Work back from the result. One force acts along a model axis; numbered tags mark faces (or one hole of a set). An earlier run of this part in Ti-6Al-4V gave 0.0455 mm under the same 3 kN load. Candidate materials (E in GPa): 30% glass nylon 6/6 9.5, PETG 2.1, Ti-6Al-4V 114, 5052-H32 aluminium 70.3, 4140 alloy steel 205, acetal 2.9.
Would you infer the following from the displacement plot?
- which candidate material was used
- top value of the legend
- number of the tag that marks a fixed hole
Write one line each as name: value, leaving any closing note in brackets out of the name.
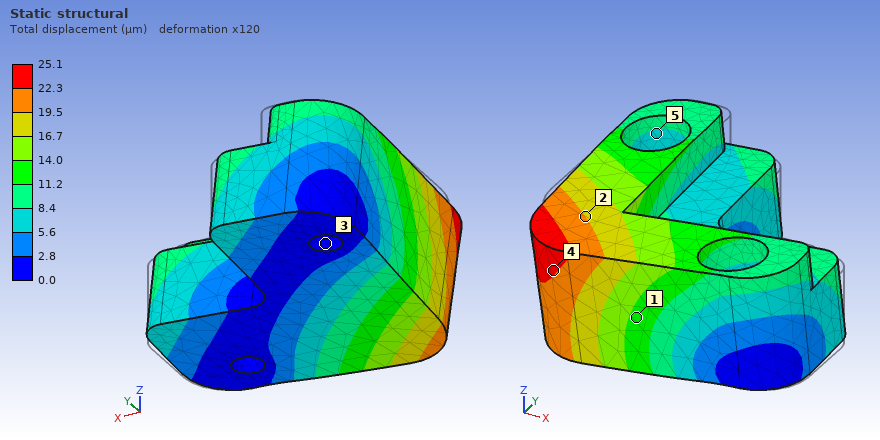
which candidate material was used: 4140 alloy steel
top value of the legend: 25.1 µm
number of the tag that marks a fixed hole: 3
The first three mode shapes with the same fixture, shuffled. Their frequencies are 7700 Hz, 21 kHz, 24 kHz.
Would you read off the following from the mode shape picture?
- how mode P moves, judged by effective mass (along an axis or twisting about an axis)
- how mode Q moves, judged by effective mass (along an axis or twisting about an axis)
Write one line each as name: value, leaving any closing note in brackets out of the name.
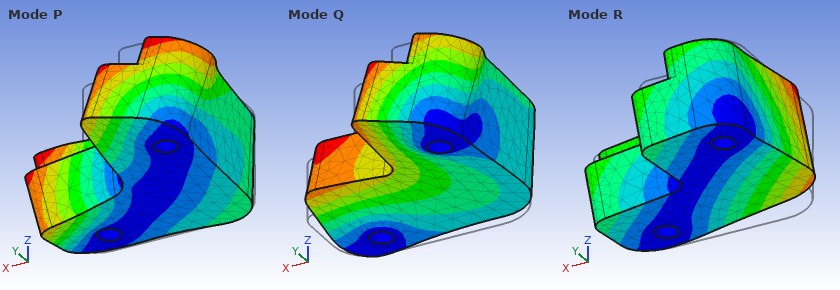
how mode P moves, judged by effective mass: twisting about Z
how mode Q moves, judged by effective mass: along Z
